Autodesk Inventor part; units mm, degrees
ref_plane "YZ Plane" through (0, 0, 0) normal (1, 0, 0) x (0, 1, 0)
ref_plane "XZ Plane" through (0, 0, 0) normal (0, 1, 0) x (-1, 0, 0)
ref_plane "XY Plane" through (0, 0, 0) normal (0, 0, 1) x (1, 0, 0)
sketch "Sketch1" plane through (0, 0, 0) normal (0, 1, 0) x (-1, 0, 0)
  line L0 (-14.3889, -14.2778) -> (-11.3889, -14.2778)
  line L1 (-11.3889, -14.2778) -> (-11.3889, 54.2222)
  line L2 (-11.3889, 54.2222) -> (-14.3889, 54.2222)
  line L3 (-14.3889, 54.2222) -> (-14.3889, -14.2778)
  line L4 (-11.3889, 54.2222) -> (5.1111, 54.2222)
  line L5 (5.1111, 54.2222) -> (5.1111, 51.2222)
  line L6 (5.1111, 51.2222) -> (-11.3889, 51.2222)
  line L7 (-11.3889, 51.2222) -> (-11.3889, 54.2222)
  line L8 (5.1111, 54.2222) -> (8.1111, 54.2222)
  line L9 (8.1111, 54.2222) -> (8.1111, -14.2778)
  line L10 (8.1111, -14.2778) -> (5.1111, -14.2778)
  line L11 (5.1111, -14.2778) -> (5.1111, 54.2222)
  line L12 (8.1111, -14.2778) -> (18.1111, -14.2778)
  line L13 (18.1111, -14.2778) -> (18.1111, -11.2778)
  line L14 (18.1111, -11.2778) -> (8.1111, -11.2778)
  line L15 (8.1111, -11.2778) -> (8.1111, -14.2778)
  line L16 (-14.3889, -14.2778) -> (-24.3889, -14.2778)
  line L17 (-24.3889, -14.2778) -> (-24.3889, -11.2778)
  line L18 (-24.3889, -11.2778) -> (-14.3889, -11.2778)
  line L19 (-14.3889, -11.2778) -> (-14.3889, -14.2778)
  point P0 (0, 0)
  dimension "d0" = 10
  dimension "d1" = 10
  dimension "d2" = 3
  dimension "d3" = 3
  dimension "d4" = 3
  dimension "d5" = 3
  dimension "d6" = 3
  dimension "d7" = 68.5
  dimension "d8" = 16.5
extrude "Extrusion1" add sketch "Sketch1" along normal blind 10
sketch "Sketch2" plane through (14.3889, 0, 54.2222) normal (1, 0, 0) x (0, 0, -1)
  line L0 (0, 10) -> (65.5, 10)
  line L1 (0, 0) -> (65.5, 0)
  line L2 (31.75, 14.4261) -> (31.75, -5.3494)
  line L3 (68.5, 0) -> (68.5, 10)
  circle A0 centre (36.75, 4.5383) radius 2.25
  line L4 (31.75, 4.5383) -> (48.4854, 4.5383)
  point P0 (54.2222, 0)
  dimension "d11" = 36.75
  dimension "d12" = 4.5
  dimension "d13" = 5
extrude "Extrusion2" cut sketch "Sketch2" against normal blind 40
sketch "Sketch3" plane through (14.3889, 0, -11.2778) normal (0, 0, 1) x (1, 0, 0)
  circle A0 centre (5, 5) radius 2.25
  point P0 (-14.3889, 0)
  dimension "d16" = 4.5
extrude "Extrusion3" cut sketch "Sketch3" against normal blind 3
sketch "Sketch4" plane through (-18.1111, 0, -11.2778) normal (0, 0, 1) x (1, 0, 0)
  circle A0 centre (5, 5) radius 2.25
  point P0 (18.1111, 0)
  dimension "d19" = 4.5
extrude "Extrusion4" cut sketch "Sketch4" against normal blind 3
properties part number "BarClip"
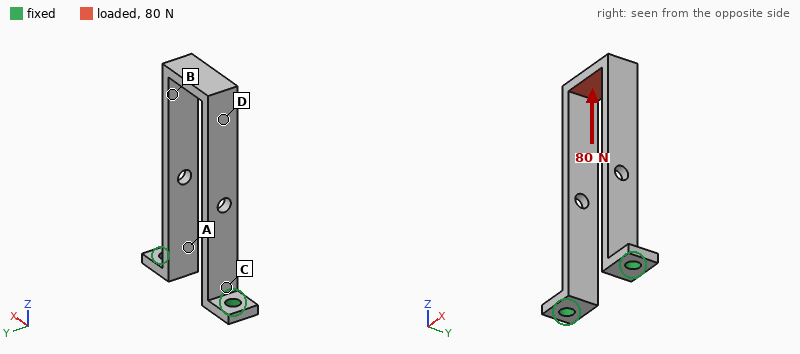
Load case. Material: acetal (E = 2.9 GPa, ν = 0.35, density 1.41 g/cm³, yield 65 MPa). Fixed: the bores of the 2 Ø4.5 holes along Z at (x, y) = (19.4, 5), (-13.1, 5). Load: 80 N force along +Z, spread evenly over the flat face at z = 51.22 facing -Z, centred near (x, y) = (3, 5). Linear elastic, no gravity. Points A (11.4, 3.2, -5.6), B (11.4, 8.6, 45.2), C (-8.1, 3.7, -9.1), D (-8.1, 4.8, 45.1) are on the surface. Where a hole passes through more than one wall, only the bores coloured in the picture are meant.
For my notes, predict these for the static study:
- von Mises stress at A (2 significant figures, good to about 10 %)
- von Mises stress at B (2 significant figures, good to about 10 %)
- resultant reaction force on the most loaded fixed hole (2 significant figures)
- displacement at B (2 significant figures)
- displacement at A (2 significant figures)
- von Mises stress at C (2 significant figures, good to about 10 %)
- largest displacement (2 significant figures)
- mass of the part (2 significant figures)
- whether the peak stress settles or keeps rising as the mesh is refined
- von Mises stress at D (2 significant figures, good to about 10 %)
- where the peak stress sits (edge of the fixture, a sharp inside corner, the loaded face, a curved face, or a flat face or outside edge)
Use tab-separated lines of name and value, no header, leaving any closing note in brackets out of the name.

von Mises stress at A	1.00 MPa
von Mises stress at B	4.8 MPa
resultant reaction force on the most loaded fixed hole	40 N
displacement at B	0.099 mm
displacement at A	0.033 mm
von Mises stress at C	4.1 MPa
largest displacement	0.15 mm
mass of the part	7.1 g
whether the peak stress settles or keeps rising as the mesh is refined	keeps rising
von Mises stress at D	2.0 MPa
where the peak stress sits	edge of the fixture
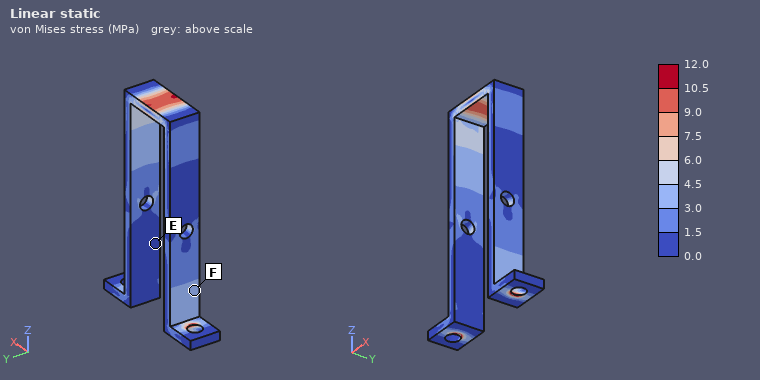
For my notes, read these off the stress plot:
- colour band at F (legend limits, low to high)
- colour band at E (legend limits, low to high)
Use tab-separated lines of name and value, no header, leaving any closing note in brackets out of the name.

colour band at F	3.0 to 4.5 MPa
colour band at E	0.0 to 1.5 MPa
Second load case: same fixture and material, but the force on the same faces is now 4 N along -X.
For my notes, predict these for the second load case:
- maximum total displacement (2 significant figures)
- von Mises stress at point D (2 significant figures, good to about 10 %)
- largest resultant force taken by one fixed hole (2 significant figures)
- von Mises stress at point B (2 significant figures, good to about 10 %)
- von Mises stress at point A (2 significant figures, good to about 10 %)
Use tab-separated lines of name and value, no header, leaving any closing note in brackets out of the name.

maximum total displacement	0.86 mm
von Mises stress at point D	3.1 MPa
largest resultant force taken by one fixed hole	6.8 N
von Mises stress at point B	3.6 MPa
von Mises stress at point A	3.0 MPa
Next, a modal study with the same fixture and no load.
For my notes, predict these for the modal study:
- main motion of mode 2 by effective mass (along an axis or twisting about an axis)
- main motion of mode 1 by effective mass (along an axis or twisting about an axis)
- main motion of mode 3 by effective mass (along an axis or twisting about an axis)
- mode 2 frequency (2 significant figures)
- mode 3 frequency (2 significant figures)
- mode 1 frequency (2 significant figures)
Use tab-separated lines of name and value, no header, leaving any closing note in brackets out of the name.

main motion of mode 2 by effective mass	along Y
main motion of mode 1 by effective mass	along X
main motion of mode 3 by effective mass	twisting about Z
mode 2 frequency	270 Hz
mode 3 frequency	610 Hz
mode 1 frequency	200 Hz
